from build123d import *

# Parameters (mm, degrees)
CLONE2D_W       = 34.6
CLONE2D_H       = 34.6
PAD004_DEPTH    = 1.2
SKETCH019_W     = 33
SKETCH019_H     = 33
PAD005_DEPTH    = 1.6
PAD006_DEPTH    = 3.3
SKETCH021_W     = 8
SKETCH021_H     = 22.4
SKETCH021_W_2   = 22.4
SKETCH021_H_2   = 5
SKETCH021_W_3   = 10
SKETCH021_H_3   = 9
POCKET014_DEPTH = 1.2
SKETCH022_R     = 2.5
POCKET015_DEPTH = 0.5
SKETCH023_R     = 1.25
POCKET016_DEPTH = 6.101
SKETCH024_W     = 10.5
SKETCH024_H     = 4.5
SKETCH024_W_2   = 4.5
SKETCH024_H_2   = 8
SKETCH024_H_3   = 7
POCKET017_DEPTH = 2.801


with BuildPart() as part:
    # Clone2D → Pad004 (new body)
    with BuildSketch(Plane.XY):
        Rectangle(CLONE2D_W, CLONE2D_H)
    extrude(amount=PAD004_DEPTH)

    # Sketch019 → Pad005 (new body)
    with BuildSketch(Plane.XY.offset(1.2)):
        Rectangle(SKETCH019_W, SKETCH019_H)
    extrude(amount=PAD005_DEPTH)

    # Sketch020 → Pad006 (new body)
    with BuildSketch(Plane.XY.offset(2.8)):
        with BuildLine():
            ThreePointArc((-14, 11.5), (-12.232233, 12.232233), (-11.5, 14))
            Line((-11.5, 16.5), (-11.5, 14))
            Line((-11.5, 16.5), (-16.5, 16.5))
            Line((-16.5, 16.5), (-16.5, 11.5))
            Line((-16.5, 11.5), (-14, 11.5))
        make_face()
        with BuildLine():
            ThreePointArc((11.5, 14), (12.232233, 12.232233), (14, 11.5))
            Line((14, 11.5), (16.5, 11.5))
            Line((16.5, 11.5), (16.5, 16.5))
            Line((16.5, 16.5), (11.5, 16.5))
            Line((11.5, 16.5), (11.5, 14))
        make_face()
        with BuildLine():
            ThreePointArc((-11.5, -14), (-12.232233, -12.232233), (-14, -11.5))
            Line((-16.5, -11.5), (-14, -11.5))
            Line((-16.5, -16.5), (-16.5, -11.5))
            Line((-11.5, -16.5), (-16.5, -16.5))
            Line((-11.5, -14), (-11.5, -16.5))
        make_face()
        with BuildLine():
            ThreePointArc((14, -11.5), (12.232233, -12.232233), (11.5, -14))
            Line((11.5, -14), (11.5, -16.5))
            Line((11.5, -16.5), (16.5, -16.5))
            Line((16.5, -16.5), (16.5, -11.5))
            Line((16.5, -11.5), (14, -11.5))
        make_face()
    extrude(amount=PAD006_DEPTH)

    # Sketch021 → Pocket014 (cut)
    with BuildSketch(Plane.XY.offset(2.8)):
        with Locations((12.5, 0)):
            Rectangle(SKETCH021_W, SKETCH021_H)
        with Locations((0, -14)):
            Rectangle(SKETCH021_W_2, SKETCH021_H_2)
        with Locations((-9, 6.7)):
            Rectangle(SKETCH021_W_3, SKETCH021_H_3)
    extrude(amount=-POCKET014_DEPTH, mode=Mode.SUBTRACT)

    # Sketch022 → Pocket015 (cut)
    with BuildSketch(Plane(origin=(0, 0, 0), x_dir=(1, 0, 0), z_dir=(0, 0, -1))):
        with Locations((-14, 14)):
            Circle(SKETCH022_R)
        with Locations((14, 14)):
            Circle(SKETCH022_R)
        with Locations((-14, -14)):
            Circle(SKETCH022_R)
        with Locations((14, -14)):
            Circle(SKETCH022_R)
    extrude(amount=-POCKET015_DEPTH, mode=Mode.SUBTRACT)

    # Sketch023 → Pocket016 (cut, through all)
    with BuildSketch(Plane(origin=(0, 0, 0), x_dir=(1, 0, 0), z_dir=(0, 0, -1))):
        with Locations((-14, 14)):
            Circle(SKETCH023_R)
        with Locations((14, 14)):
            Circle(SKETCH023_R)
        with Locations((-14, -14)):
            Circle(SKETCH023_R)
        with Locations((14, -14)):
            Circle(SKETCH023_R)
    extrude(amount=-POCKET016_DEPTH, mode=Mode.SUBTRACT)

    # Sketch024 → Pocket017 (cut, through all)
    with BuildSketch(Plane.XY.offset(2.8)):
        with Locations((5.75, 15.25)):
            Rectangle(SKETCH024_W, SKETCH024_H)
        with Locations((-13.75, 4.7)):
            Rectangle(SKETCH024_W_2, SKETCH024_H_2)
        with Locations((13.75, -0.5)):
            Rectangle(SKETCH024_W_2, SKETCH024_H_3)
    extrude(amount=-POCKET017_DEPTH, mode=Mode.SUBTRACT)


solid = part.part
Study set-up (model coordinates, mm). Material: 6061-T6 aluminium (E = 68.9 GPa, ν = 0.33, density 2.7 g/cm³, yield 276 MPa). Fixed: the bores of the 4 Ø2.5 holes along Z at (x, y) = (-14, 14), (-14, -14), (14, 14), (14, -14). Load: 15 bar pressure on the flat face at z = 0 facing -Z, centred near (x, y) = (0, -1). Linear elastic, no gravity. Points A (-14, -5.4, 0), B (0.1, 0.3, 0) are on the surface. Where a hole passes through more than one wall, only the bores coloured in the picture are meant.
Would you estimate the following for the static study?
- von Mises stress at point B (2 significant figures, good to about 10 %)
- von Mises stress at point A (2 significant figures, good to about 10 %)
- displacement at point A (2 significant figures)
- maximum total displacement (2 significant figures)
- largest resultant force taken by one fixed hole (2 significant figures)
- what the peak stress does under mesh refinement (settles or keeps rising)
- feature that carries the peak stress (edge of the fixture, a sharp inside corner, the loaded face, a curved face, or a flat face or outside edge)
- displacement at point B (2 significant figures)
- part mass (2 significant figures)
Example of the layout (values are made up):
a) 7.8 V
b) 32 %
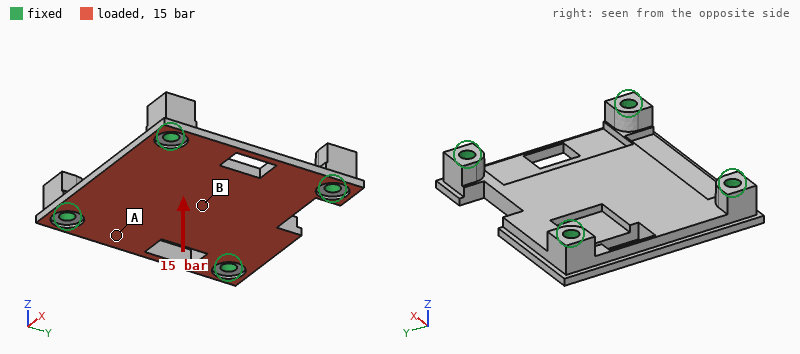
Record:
a) 53 MPa
b) 24 MPa
c) 26 µm
d) 73 µm
e) 460 N
f) keeps rising
g) a sharp inside corner
h) 73 µm
i) 7.1 g
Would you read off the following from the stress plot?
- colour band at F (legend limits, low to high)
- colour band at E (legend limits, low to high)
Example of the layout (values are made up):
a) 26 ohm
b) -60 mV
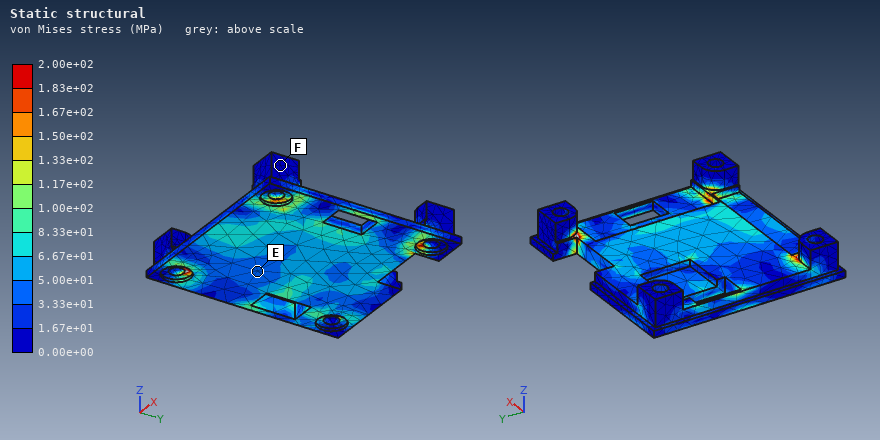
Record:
a) 0.00e+00 to 1.67e+01 MPa
b) 3.33e+01 to 5.00e+01 MPa
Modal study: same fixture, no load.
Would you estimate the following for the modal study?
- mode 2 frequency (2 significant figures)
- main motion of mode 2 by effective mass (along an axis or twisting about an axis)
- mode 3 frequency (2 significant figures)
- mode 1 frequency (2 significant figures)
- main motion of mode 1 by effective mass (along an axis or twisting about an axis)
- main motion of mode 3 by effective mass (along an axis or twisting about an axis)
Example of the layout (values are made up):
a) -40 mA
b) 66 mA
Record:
a) 17 kHz
b) twisting about X
c) 18 kHz
d) 10 kHz
e) along Z
f) twisting about Y
